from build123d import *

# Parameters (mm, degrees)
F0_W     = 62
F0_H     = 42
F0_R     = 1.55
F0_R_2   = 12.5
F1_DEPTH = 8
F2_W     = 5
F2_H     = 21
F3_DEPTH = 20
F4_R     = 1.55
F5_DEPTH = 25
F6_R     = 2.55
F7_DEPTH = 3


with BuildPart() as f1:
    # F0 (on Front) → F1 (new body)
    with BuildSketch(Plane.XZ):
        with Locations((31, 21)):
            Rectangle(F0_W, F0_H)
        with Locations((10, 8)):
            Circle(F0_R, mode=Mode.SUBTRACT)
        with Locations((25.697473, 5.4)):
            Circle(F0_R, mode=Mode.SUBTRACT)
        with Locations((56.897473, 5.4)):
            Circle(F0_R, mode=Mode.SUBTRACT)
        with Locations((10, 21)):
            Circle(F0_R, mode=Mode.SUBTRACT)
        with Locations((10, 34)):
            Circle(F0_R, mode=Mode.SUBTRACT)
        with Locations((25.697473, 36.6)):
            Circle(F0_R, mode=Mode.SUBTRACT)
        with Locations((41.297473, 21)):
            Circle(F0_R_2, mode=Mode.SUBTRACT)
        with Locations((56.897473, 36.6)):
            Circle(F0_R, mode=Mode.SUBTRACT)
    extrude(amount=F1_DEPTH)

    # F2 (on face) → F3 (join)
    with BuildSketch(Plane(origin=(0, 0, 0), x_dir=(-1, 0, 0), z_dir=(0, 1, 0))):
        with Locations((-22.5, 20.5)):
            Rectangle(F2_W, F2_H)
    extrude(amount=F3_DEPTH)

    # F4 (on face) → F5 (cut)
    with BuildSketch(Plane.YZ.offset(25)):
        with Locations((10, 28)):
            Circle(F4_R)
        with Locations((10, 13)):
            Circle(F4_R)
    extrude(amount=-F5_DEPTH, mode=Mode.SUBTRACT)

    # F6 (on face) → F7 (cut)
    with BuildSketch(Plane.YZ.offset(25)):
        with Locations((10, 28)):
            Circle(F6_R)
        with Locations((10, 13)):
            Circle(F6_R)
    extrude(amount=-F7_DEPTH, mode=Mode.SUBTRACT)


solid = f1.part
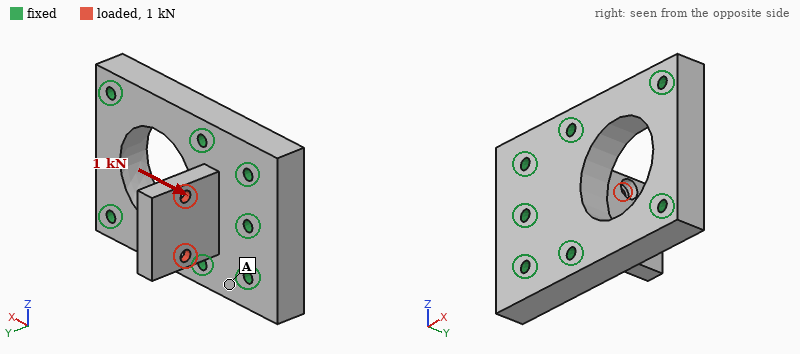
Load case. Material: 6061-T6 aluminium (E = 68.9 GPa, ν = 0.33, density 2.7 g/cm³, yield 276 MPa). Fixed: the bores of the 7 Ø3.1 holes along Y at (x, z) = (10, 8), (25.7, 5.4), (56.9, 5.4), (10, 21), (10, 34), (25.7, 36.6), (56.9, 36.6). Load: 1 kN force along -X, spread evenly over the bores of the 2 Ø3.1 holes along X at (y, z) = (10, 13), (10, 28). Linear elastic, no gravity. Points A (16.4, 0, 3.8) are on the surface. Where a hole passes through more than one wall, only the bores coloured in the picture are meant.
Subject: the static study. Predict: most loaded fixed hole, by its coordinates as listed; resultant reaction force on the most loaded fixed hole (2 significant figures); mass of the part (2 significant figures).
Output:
(10, 21)
520 N
50 g
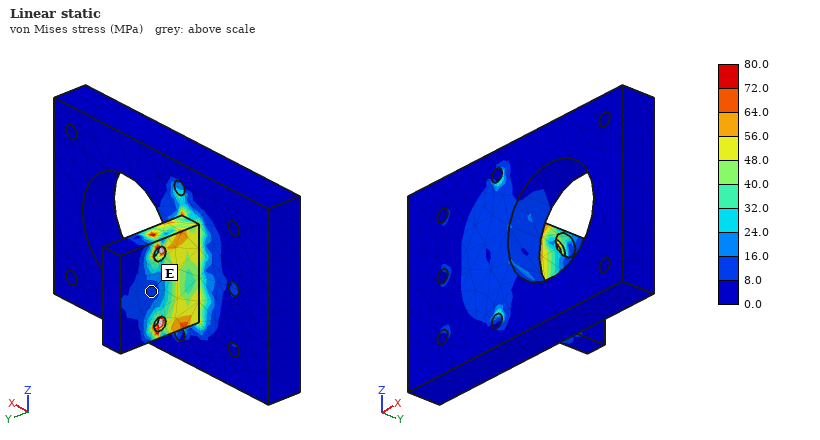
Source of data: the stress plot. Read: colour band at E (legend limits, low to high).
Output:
8.0 to 16.0 MPa
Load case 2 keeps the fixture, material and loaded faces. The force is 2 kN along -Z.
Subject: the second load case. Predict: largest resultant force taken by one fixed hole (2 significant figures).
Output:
1.1 kN
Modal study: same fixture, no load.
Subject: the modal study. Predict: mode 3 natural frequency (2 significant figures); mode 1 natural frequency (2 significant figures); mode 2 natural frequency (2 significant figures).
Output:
20 kHz
8200 Hz
18 kHz
